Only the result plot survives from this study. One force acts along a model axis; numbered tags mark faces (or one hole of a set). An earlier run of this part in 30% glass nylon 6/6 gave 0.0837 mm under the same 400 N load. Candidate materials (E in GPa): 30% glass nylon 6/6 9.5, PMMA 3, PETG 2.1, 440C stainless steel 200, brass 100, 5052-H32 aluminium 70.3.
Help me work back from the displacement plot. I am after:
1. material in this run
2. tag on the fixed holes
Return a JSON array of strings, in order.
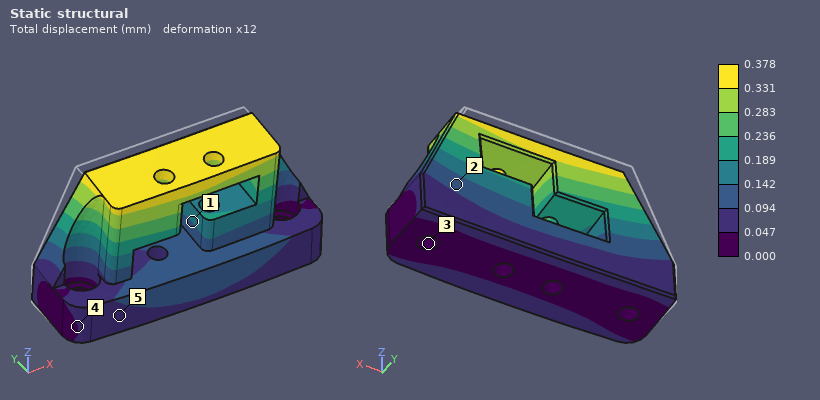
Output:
["PETG", "3"]
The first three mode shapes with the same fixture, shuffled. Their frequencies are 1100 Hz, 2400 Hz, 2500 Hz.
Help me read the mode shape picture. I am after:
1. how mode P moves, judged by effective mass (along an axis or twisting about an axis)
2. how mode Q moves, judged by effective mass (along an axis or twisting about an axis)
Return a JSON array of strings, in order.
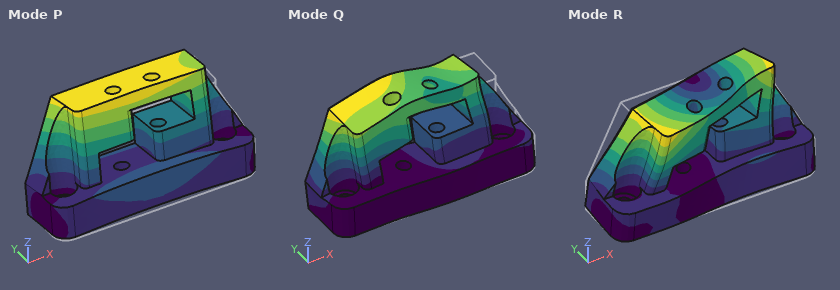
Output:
["along Y", "along X"]
